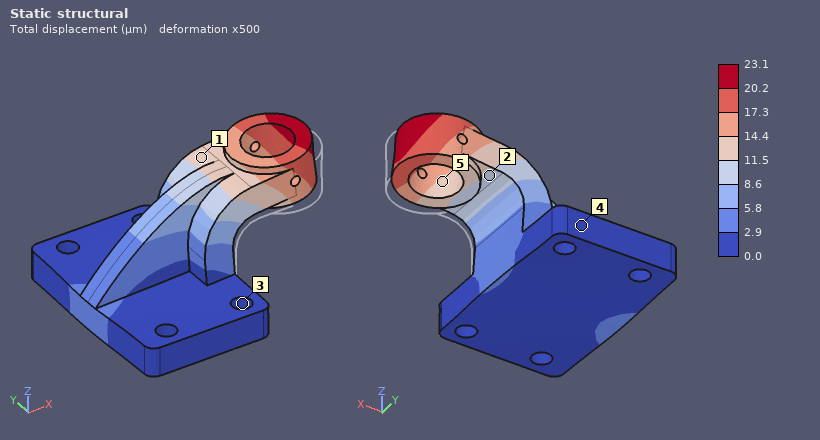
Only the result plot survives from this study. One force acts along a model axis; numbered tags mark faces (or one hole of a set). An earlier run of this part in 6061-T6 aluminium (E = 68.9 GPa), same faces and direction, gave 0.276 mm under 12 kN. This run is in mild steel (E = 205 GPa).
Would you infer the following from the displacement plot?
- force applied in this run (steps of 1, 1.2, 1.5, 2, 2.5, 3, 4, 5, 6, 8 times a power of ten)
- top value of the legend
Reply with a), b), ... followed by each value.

a) 3 kN
b) 23.1 µm
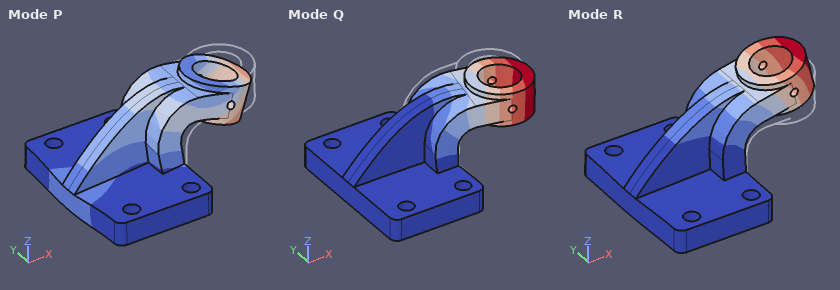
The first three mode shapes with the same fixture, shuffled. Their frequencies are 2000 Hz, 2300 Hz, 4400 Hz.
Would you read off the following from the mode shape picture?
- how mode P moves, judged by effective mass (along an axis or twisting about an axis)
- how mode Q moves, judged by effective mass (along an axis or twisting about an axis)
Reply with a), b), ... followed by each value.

a) along X
b) along Y
